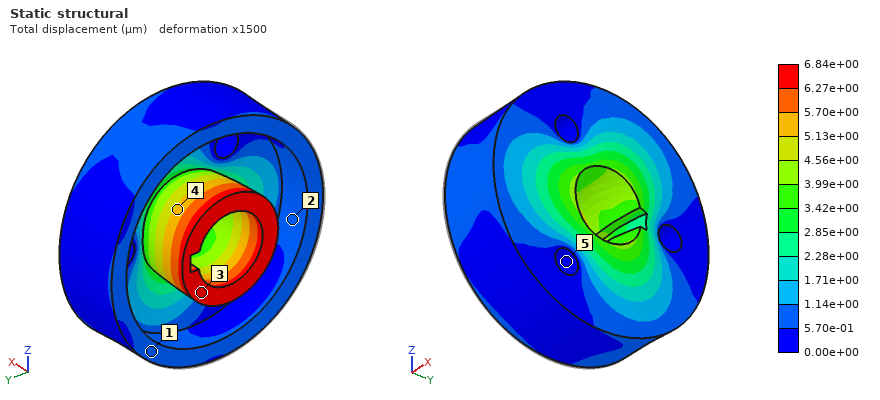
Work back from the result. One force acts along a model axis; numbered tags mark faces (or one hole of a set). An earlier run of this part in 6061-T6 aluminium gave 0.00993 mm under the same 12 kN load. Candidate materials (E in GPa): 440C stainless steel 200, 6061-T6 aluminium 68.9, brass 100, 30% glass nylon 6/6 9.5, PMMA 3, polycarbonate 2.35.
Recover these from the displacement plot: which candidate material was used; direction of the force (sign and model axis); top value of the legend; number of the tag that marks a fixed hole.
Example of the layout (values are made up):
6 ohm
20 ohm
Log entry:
brass
+X
6.84e+00 µm
5
